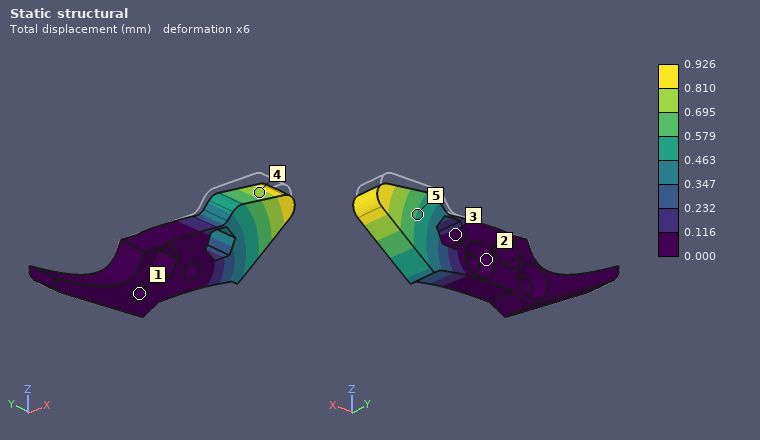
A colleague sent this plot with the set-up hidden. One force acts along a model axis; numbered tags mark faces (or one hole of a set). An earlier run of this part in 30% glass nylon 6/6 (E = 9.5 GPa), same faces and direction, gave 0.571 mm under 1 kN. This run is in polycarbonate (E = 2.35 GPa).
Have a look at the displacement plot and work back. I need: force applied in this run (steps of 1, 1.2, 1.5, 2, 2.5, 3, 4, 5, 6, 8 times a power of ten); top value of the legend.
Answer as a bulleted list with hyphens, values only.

- 400 N
- 0.926 mm
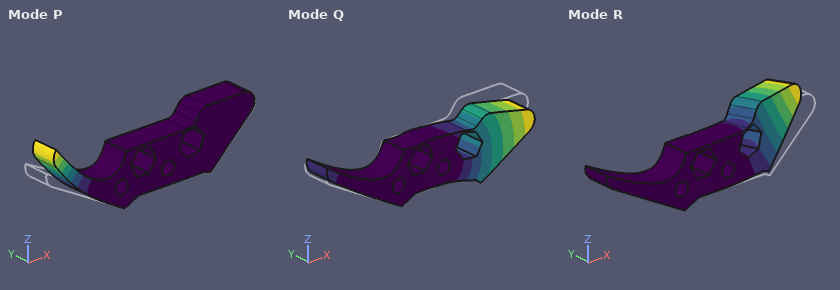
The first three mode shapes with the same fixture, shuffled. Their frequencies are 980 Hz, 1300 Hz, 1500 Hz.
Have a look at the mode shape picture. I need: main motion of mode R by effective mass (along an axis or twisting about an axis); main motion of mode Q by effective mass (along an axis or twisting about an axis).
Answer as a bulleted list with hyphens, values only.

- along Y
- along Z
